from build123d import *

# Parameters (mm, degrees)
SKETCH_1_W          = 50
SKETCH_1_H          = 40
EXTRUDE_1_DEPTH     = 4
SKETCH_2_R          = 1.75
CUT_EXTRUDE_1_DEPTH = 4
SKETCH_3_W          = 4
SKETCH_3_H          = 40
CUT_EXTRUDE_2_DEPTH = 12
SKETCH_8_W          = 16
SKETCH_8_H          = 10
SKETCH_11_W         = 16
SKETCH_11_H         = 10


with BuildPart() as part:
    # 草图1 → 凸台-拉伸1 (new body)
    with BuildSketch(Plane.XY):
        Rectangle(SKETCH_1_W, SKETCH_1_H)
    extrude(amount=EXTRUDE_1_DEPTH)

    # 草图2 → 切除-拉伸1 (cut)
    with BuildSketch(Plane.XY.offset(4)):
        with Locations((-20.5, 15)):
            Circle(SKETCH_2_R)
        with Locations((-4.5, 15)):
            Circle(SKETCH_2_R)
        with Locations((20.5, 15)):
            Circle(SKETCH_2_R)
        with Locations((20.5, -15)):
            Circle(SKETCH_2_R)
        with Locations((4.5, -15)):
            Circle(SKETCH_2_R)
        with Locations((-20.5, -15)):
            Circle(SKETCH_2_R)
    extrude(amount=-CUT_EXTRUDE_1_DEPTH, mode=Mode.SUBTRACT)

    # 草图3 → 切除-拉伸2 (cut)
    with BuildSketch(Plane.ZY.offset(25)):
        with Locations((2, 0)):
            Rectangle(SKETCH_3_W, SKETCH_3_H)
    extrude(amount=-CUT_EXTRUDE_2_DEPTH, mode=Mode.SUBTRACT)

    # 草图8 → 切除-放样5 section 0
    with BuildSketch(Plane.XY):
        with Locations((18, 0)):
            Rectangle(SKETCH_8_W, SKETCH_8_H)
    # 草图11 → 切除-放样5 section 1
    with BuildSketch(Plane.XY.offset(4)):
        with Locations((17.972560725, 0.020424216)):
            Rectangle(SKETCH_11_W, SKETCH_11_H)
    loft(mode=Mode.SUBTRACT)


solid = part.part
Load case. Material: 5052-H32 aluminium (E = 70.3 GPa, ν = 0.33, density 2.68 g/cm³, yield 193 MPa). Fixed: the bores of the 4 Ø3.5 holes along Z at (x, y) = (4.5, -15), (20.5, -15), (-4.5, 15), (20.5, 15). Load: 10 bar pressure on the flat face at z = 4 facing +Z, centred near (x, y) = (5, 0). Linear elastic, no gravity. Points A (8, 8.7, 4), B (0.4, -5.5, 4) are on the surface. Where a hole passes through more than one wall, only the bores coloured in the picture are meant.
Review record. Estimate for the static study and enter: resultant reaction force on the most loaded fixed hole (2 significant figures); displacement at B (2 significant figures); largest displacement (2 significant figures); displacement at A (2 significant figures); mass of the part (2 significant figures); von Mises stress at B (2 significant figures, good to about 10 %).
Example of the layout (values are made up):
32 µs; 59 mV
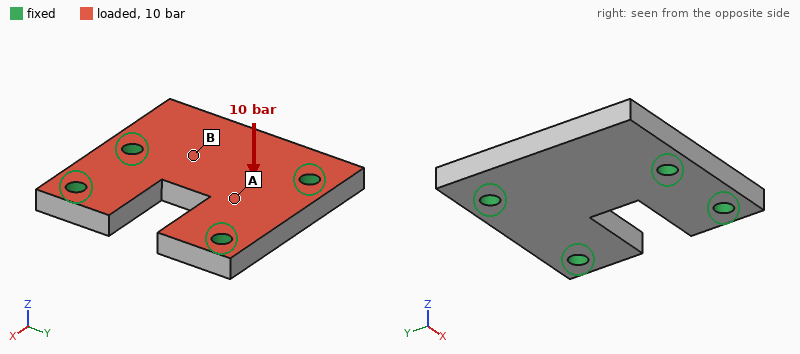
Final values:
490 N; 9.1 µm; 27 µm; 5.7 µm; 14 g; 19 MPa
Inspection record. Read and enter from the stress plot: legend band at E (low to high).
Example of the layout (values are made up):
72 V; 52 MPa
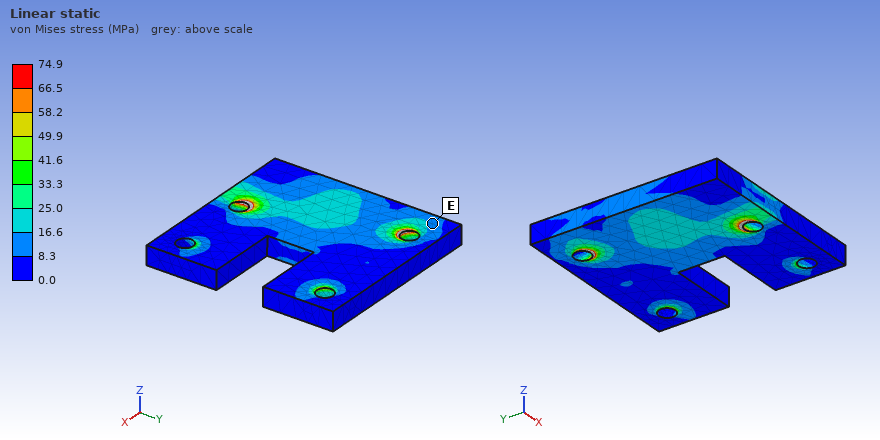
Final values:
8.3 to 16.6 MPa
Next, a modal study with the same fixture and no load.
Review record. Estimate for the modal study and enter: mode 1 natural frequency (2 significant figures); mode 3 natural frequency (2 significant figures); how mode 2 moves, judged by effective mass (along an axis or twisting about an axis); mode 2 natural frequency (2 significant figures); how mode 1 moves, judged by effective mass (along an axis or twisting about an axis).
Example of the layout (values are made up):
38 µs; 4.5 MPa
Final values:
12 kHz; 25 kHz; along Z; 20 kHz; along Z
